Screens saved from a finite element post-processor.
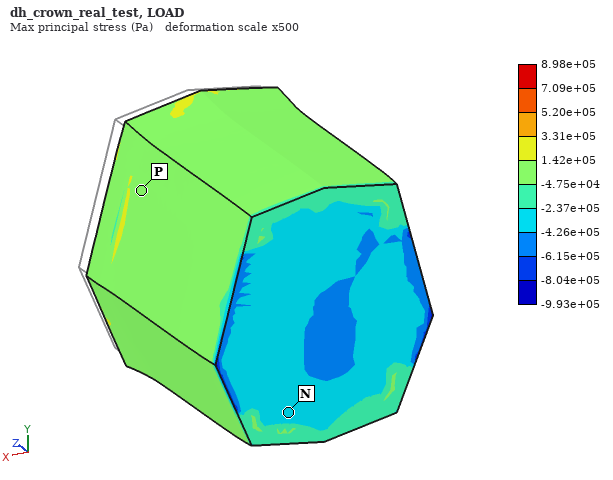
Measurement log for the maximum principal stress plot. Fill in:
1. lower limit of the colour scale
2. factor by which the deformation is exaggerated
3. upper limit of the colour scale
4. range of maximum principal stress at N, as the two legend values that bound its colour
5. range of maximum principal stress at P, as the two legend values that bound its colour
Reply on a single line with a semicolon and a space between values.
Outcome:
-9.93e+05 Pa; 500; 8.98e+05 Pa; -4.26e+05 to -2.37e+05 Pa; -4.75e+04 to 1.42e+05 Pa
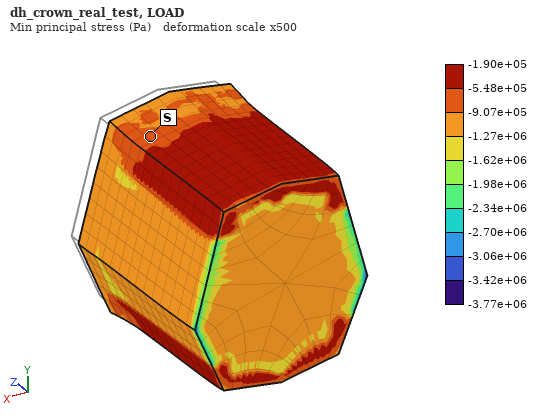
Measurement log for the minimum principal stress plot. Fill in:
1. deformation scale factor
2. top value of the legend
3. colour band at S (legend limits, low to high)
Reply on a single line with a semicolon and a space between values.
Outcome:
500; -1.90e+05 Pa; -9.07e+05 to -5.48e+05 Pa
